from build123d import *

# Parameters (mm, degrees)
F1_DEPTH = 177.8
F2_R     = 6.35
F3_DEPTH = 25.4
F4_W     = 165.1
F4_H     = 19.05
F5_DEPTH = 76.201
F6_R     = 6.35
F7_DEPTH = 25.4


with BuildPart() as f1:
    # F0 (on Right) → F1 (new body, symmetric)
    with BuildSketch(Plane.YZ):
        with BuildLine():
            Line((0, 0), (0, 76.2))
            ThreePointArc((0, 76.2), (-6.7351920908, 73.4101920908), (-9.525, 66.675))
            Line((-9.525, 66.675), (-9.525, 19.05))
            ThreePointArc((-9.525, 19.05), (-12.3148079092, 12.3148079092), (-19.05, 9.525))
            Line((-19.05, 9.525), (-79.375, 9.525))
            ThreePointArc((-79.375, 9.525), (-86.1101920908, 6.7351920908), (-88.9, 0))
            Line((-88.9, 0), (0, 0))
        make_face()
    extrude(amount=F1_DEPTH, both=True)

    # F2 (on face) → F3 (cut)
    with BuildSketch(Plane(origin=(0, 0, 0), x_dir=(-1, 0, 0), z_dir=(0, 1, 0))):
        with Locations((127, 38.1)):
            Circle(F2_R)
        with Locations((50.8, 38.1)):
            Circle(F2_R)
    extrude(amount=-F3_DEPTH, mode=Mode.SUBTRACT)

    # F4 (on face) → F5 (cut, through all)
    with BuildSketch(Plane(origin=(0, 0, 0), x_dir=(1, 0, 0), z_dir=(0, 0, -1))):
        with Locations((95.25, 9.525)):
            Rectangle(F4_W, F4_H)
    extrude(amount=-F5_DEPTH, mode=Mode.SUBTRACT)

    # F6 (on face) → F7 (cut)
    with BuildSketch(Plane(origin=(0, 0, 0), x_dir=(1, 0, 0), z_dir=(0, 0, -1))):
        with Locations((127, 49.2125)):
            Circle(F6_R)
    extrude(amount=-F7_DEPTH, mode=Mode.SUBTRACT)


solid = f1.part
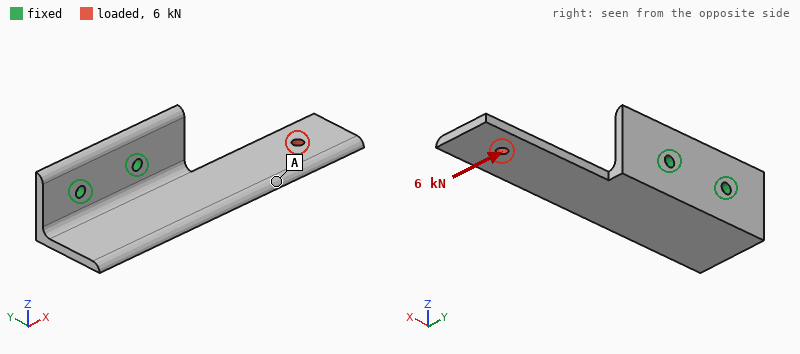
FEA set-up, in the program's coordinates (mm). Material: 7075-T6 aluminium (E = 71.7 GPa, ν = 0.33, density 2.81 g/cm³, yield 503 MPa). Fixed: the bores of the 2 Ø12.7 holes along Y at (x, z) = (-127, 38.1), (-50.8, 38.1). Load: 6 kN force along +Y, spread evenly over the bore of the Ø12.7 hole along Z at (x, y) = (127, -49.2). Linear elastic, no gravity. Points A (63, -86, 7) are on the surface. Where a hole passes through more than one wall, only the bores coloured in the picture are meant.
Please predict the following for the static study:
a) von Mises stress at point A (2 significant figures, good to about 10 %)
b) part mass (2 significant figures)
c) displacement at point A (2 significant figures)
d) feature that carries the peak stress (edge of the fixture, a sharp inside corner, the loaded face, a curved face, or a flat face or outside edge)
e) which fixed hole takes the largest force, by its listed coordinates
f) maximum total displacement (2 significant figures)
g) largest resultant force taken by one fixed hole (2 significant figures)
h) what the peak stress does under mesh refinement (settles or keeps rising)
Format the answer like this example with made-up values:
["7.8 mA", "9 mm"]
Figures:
["52 MPa", "1.1 kg", "1.9 mm", "edge of the fixture", "(-50.8, 38.1)", "3.3 mm", "17 kN", "keeps rising"]
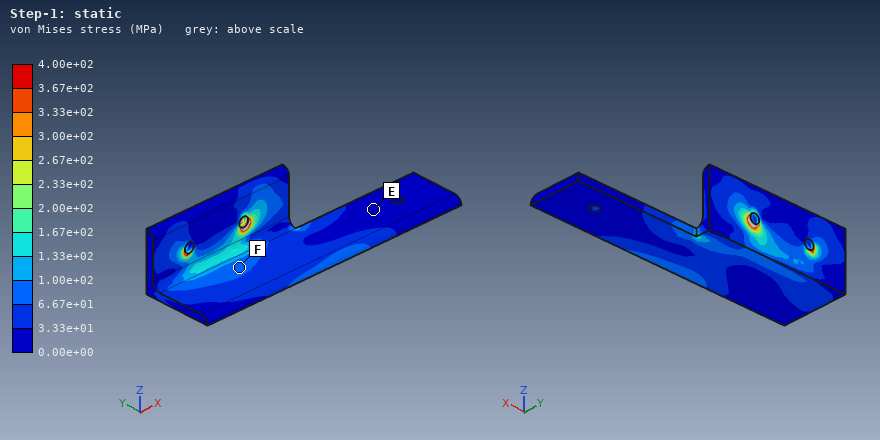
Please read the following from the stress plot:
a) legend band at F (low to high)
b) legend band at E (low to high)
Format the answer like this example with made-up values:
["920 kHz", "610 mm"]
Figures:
["6.67e+01 to 1.00e+02 MPa", "0.00e+00 to 3.33e+01 MPa"]
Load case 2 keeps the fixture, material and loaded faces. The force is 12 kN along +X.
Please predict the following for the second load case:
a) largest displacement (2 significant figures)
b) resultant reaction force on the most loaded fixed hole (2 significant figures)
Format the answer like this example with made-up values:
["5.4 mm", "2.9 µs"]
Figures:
["0.88 mm", "9.8 kN"]
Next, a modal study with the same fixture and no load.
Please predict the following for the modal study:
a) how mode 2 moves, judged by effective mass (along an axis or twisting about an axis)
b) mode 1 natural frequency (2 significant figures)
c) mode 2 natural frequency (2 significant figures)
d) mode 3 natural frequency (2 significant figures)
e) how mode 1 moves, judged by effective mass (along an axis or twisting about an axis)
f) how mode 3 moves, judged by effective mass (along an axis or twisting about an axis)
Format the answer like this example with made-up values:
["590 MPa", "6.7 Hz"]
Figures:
["along Y", "190 Hz", "500 Hz", "680 Hz", "along Z", "along Z"]
